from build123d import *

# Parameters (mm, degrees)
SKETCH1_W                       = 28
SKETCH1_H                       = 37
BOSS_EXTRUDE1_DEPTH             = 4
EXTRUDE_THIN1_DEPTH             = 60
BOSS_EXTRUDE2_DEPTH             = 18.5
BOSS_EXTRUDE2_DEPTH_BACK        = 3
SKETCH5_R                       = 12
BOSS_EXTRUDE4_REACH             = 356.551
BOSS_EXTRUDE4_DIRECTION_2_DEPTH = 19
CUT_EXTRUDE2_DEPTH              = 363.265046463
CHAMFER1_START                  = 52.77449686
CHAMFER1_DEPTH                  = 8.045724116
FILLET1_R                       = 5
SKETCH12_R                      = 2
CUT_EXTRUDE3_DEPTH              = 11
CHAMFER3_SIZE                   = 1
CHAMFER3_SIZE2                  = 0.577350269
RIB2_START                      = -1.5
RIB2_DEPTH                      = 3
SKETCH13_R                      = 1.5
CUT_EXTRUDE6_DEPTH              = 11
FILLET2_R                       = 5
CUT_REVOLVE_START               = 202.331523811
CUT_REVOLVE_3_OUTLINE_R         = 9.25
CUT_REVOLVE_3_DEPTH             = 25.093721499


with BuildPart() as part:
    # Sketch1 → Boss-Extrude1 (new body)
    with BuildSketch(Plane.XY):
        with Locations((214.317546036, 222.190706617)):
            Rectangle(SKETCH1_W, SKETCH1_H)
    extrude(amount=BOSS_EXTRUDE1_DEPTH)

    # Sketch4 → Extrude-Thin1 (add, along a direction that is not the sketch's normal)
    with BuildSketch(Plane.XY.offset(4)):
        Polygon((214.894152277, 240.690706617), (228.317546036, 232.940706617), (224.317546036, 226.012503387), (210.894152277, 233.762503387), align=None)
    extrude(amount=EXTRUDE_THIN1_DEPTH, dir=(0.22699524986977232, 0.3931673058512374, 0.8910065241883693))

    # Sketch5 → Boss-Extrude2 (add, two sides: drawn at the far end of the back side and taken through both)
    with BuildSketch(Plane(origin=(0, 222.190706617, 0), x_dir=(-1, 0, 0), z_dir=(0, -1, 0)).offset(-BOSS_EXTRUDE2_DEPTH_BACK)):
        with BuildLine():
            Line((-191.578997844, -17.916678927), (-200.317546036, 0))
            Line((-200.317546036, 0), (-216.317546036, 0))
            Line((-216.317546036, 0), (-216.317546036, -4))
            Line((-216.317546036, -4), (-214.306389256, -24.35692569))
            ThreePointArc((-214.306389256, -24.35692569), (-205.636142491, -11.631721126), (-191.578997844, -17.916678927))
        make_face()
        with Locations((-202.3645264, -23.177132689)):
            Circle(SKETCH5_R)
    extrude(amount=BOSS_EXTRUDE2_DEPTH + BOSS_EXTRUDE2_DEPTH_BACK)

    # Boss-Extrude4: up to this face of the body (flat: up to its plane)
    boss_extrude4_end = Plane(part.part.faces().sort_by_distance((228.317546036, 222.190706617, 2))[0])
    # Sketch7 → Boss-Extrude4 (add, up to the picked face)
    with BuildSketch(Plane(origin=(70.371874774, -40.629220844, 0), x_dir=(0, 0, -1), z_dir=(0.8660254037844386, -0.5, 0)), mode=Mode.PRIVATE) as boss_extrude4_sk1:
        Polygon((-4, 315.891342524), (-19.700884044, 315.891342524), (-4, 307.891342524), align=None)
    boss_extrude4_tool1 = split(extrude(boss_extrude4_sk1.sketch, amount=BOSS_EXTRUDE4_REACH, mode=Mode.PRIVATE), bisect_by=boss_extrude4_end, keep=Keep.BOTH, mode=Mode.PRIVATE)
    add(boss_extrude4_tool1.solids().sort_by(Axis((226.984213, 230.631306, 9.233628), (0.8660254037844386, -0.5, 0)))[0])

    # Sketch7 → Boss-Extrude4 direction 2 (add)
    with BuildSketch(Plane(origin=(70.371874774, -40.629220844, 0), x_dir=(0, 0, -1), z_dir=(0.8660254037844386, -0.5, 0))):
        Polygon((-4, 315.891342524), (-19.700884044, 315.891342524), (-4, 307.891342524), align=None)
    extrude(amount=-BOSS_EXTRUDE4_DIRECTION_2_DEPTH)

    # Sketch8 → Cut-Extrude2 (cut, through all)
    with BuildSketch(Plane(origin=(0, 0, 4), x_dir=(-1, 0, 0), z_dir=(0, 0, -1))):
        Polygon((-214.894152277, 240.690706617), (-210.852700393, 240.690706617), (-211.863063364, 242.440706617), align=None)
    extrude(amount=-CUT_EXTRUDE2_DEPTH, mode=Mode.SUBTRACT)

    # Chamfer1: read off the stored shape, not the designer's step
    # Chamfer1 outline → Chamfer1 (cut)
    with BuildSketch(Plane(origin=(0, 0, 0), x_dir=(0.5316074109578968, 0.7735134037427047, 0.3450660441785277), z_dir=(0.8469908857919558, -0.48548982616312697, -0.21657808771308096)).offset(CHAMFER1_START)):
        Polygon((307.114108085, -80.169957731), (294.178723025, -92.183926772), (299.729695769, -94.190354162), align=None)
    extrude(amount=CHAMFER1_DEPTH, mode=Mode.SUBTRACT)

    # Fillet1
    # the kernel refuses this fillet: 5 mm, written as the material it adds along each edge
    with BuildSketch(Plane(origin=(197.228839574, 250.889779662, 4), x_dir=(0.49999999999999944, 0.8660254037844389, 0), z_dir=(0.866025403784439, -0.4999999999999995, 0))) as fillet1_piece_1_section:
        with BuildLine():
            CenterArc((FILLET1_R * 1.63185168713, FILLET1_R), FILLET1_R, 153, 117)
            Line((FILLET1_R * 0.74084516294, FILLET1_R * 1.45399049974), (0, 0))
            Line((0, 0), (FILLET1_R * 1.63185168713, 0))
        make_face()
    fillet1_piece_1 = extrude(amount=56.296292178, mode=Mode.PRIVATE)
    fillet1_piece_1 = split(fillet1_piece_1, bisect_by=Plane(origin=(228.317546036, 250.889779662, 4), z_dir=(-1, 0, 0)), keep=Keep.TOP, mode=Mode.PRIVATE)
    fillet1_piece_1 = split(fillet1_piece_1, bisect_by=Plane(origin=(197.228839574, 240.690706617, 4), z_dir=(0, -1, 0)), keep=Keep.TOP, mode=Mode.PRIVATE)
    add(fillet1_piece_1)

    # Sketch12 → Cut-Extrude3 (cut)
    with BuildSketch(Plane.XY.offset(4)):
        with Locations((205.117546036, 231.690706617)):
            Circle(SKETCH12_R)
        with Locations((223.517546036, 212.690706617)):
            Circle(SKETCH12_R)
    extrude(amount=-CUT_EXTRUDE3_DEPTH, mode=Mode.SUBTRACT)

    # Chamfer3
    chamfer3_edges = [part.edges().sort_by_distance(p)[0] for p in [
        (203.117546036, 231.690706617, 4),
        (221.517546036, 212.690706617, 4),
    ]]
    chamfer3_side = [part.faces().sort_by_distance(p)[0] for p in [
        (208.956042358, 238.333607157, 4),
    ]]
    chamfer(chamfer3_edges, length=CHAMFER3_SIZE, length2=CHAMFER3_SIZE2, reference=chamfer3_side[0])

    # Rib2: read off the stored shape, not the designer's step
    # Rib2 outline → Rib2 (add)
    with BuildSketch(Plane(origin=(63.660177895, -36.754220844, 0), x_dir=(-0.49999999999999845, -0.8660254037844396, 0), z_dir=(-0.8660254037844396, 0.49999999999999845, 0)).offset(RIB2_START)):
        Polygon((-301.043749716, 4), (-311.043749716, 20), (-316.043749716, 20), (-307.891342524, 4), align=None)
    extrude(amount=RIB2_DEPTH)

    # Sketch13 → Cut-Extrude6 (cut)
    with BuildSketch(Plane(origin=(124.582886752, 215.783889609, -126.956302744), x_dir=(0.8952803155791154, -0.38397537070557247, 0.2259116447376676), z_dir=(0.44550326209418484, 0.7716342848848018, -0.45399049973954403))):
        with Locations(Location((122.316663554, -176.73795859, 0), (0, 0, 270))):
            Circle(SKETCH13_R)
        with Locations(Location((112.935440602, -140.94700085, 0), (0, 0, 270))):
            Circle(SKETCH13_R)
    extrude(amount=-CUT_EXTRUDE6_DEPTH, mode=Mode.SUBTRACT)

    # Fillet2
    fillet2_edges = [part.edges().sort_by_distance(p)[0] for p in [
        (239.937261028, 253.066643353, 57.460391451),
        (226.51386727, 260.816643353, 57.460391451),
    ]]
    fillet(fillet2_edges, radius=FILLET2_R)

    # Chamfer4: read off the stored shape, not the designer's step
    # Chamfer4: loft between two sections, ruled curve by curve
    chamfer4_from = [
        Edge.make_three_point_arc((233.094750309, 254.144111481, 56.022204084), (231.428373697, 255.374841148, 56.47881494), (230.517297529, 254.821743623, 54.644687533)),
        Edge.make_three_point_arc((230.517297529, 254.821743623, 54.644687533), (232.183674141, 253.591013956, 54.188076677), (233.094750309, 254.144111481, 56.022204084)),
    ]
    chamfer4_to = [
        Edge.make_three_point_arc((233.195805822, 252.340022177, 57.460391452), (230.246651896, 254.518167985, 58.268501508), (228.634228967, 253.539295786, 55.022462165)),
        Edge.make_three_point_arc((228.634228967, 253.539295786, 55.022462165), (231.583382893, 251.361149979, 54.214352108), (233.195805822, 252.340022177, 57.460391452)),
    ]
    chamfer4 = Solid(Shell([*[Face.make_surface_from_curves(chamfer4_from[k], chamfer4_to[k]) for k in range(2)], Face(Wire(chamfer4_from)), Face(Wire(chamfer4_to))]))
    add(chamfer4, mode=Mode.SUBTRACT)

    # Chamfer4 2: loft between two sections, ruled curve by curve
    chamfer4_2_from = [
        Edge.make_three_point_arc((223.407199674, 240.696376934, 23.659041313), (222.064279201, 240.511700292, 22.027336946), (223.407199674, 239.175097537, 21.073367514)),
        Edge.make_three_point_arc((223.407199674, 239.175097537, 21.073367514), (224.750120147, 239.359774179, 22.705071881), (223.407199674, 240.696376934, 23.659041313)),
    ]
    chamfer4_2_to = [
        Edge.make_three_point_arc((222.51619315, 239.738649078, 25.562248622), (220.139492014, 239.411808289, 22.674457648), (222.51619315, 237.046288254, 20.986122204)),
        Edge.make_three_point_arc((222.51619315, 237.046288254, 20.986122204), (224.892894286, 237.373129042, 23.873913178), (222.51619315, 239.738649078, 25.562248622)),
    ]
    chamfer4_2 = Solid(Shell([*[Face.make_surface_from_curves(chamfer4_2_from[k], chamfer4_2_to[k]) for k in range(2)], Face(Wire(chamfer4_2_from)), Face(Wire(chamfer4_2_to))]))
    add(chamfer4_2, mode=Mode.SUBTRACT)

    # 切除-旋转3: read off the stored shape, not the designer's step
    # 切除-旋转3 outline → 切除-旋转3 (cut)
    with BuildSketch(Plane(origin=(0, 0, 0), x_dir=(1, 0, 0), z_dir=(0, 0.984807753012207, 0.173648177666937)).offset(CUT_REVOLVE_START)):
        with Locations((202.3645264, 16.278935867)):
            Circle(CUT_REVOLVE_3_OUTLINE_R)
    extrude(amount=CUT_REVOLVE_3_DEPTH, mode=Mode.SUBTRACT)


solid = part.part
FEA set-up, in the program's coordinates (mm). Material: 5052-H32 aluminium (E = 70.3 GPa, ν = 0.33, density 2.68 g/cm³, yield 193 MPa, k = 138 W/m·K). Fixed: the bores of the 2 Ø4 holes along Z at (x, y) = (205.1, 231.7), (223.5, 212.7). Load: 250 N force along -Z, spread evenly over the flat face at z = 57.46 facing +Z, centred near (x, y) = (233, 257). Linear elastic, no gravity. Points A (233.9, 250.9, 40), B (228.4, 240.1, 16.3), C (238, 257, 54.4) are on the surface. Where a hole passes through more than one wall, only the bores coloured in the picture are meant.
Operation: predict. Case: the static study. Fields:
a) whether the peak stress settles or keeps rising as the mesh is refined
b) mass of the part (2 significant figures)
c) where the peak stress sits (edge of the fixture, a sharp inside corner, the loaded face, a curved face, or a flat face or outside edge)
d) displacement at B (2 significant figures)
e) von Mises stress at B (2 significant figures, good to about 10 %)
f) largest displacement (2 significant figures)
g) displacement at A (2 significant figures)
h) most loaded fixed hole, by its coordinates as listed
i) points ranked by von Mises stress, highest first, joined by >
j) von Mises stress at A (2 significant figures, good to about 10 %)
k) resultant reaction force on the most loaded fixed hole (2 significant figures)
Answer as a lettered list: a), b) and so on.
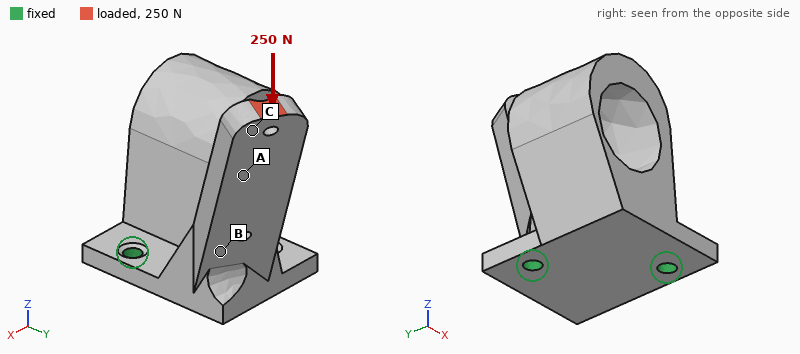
a) keeps rising
b) 51 g
c) edge of the fixture
d) 0.13 mm
e) 41 MPa
f) 0.51 mm
g) 0.33 mm
h) (205.1, 231.7)
i) B > A > C
j) 18 MPa
k) 240 N
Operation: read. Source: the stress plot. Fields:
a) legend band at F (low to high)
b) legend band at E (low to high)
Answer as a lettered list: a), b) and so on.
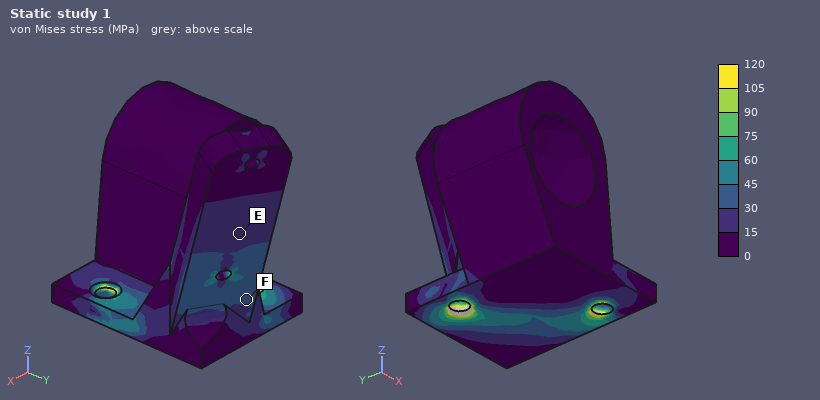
a) 30 to 45 MPa
b) 15 to 30 MPa
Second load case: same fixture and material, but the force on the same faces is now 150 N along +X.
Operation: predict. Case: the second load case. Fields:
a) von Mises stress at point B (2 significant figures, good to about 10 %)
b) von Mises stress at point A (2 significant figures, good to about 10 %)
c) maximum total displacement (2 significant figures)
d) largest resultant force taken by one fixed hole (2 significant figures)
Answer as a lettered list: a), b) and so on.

a) 33 MPa
b) 13 MPa
c) 0.36 mm
d) 350 N
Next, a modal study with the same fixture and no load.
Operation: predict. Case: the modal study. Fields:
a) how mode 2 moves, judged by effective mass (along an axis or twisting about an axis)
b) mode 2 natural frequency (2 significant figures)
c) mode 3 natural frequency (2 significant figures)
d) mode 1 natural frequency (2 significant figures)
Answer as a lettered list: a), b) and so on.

a) along X
b) 2300 Hz
c) 2900 Hz
d) 1100 Hz
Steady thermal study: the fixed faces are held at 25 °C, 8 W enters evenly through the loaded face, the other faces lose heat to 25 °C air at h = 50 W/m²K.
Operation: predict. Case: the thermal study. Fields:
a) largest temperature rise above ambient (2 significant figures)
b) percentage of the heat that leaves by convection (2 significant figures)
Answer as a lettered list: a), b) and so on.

a) 35 K
b) 33 %
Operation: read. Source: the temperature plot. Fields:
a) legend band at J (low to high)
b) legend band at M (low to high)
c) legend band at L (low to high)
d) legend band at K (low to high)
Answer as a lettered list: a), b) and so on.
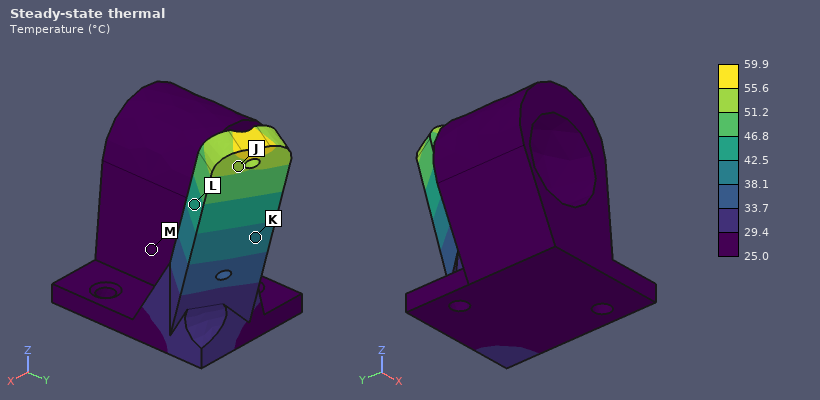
a) 51.2 to 55.6 °C
b) 25.0 to 29.4 °C
c) 42.5 to 46.8 °C
d) 38.1 to 42.5 °C
